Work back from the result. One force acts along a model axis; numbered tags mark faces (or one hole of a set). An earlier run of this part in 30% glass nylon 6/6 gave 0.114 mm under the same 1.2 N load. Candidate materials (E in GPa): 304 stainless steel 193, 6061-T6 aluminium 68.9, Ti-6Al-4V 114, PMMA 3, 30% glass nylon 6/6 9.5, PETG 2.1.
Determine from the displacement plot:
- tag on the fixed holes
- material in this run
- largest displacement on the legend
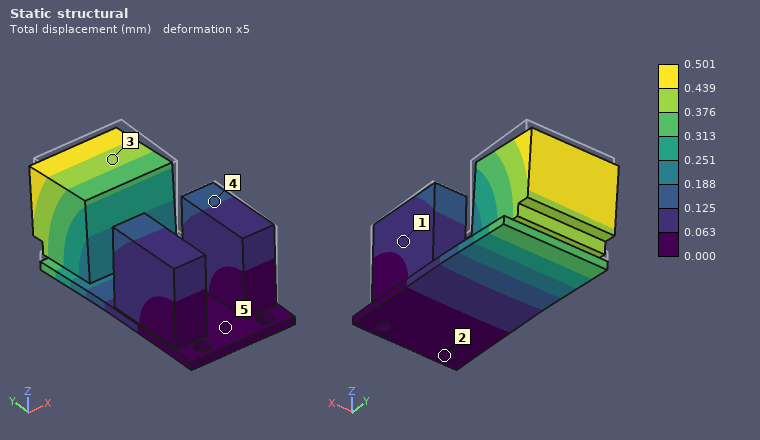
2
PETG
0.501 mm
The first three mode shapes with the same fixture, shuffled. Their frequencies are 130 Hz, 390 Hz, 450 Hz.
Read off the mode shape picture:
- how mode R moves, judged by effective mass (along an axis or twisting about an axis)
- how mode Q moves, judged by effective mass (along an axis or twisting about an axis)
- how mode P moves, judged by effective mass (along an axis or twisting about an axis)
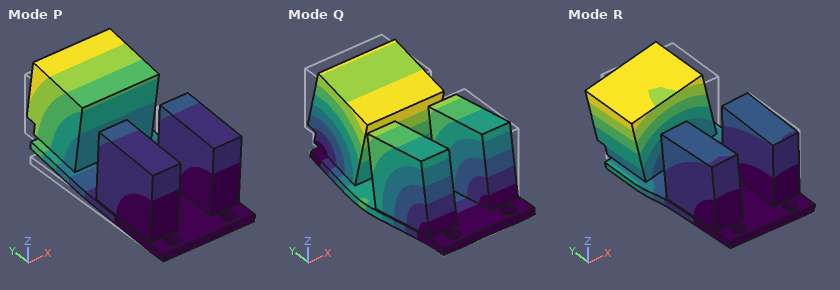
along X
along Z
along Z
